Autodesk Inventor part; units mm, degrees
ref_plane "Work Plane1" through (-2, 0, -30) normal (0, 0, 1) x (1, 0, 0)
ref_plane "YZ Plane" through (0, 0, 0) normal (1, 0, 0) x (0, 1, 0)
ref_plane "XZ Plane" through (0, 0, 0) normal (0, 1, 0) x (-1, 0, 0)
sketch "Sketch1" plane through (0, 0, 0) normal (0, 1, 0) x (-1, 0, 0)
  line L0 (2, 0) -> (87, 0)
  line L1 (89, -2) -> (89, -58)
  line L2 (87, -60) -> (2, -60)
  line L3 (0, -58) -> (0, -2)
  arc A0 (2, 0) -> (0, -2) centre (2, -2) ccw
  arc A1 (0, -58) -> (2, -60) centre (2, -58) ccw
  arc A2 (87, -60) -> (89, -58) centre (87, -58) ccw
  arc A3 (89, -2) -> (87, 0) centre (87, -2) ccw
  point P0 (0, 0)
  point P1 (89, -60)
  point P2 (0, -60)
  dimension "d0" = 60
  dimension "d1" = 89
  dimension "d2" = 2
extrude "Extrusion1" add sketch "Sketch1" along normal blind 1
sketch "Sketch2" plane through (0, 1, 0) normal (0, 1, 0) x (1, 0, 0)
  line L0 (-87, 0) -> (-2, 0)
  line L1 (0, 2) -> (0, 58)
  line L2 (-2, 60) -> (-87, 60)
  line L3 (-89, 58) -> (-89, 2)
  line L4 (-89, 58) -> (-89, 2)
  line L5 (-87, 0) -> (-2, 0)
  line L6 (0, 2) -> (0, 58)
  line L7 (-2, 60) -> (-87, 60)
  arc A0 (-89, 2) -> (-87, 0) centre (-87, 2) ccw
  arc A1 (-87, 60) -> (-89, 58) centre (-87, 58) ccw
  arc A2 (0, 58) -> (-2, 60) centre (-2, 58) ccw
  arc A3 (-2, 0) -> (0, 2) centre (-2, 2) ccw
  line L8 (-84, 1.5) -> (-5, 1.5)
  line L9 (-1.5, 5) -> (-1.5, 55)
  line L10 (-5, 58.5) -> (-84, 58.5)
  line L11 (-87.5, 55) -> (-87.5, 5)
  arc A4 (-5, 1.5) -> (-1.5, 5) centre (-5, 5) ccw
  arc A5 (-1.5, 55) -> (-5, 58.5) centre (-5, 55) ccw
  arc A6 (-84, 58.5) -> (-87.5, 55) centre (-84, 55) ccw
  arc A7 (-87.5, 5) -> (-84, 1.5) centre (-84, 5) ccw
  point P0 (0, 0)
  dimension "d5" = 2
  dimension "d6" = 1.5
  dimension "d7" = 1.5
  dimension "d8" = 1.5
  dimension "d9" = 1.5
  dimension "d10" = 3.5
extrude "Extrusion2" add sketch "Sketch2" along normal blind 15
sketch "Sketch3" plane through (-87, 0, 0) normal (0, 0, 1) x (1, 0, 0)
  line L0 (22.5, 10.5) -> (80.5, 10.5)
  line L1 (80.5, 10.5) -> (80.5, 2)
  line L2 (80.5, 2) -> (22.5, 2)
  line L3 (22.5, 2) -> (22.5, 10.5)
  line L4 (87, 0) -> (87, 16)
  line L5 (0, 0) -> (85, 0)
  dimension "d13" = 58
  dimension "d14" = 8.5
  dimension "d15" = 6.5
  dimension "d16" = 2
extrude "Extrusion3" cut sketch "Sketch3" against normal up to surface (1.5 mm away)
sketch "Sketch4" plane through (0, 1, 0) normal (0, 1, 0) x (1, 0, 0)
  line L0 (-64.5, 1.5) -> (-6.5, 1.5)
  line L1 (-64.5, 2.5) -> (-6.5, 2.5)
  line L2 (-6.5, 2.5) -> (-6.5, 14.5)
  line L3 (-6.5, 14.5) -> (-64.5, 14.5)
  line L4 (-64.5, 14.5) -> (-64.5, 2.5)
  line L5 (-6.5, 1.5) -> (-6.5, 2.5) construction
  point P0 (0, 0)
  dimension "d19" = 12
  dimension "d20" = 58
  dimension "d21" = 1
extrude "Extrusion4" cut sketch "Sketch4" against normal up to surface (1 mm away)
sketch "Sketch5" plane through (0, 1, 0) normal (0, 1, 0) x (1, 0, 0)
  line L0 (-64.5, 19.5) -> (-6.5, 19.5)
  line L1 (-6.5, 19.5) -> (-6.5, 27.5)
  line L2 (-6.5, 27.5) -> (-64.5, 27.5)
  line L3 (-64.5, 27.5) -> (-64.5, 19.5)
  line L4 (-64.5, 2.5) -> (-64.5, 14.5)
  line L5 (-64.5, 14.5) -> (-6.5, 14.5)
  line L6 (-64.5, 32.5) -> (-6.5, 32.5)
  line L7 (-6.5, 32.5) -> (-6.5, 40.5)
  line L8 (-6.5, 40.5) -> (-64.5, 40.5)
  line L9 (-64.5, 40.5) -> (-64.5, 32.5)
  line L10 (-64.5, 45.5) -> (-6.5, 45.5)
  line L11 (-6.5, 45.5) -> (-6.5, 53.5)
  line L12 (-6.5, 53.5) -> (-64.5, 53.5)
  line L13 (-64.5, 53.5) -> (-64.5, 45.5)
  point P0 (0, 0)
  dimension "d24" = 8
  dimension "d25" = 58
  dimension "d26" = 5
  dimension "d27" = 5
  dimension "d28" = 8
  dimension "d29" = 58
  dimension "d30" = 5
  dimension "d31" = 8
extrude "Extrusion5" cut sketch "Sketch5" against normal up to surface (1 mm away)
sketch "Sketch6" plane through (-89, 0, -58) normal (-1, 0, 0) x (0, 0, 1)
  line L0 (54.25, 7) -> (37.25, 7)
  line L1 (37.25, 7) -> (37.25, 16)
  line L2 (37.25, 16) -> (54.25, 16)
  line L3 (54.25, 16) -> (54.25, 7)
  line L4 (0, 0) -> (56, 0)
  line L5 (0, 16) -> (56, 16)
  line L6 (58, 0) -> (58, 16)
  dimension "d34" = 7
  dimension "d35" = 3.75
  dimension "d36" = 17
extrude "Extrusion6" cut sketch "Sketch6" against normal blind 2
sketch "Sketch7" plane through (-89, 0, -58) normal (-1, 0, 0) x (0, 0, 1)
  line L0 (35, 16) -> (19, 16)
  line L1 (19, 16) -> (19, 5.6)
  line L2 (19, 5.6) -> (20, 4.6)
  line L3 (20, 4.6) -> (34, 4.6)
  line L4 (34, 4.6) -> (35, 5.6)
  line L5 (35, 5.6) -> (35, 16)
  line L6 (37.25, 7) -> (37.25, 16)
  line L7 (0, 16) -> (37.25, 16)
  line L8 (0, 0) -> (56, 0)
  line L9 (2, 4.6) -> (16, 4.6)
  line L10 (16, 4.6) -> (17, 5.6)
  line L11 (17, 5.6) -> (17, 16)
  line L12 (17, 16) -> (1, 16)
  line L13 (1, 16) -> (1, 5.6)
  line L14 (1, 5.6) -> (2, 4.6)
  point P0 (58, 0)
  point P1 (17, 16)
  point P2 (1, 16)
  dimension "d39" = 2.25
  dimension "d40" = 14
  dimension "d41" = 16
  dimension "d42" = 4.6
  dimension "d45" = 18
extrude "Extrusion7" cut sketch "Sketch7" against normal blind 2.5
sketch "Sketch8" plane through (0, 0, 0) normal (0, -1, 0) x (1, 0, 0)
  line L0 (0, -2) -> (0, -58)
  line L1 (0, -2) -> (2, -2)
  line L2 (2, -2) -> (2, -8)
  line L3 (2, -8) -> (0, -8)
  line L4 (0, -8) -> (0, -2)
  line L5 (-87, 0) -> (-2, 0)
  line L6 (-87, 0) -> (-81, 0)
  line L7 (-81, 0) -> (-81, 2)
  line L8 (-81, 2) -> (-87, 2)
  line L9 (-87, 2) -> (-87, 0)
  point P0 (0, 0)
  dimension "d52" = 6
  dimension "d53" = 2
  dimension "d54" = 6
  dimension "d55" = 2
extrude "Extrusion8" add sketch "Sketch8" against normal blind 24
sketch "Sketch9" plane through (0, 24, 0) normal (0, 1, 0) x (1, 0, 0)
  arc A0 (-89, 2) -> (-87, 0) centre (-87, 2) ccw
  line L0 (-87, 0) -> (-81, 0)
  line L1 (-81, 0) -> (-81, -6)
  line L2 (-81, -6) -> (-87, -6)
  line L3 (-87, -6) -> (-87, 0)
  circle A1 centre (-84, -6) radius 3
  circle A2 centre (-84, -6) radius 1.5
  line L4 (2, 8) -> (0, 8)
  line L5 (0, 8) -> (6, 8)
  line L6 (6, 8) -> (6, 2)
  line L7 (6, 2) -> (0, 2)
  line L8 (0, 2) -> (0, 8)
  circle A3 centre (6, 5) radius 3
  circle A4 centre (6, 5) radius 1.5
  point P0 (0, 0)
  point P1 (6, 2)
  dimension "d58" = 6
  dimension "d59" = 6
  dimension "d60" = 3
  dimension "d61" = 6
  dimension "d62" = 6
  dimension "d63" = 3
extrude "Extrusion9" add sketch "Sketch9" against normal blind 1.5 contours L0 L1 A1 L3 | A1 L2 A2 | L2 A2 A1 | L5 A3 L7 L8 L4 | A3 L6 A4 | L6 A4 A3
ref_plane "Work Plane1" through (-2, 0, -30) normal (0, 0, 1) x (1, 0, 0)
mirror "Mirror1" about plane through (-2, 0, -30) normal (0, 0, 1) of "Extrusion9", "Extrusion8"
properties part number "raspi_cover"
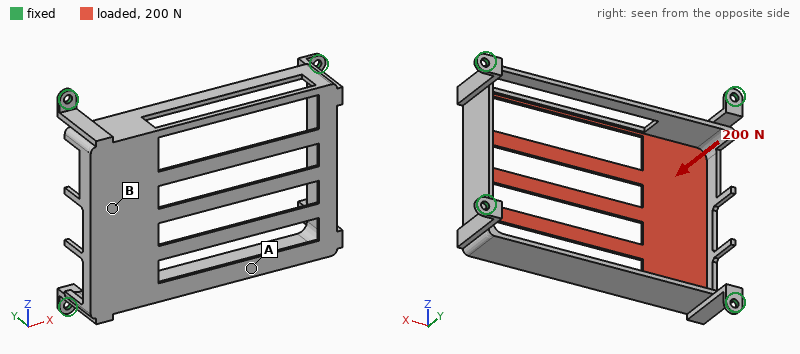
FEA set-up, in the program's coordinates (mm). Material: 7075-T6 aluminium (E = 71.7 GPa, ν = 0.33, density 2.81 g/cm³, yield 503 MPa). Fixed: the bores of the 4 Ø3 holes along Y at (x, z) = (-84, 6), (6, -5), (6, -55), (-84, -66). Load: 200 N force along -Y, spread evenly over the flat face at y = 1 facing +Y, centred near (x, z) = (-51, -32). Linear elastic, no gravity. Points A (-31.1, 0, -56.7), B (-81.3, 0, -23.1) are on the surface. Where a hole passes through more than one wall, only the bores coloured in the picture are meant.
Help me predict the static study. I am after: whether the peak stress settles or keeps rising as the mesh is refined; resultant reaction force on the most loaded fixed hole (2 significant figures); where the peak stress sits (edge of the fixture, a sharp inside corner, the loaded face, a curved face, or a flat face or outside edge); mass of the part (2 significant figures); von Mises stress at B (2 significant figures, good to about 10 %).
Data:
keeps rising
76 N
a sharp inside corner
27 g
36 MPa
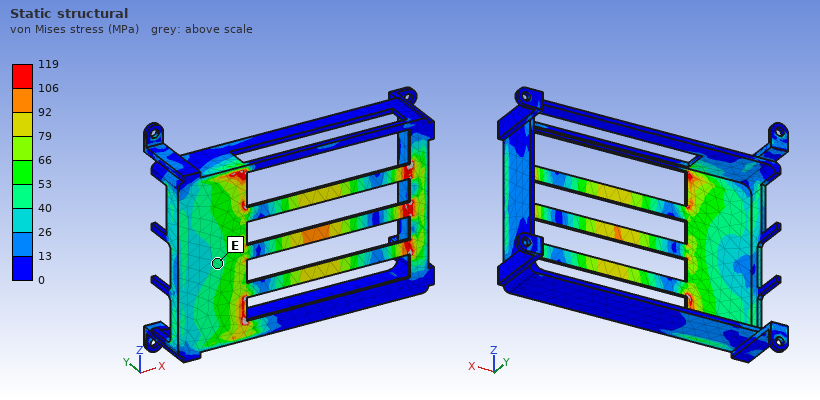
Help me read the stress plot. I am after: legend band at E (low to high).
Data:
40 to 53 MPa
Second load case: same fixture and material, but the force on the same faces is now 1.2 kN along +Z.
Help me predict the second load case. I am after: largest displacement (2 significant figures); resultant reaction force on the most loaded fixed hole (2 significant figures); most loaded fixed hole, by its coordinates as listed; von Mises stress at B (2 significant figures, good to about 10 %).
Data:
0.82 mm
450 N
(-84, 6)
60 MPa
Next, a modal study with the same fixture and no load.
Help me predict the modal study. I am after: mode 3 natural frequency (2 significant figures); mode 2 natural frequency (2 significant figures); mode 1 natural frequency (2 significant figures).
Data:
1300 Hz
1200 Hz
980 Hz
